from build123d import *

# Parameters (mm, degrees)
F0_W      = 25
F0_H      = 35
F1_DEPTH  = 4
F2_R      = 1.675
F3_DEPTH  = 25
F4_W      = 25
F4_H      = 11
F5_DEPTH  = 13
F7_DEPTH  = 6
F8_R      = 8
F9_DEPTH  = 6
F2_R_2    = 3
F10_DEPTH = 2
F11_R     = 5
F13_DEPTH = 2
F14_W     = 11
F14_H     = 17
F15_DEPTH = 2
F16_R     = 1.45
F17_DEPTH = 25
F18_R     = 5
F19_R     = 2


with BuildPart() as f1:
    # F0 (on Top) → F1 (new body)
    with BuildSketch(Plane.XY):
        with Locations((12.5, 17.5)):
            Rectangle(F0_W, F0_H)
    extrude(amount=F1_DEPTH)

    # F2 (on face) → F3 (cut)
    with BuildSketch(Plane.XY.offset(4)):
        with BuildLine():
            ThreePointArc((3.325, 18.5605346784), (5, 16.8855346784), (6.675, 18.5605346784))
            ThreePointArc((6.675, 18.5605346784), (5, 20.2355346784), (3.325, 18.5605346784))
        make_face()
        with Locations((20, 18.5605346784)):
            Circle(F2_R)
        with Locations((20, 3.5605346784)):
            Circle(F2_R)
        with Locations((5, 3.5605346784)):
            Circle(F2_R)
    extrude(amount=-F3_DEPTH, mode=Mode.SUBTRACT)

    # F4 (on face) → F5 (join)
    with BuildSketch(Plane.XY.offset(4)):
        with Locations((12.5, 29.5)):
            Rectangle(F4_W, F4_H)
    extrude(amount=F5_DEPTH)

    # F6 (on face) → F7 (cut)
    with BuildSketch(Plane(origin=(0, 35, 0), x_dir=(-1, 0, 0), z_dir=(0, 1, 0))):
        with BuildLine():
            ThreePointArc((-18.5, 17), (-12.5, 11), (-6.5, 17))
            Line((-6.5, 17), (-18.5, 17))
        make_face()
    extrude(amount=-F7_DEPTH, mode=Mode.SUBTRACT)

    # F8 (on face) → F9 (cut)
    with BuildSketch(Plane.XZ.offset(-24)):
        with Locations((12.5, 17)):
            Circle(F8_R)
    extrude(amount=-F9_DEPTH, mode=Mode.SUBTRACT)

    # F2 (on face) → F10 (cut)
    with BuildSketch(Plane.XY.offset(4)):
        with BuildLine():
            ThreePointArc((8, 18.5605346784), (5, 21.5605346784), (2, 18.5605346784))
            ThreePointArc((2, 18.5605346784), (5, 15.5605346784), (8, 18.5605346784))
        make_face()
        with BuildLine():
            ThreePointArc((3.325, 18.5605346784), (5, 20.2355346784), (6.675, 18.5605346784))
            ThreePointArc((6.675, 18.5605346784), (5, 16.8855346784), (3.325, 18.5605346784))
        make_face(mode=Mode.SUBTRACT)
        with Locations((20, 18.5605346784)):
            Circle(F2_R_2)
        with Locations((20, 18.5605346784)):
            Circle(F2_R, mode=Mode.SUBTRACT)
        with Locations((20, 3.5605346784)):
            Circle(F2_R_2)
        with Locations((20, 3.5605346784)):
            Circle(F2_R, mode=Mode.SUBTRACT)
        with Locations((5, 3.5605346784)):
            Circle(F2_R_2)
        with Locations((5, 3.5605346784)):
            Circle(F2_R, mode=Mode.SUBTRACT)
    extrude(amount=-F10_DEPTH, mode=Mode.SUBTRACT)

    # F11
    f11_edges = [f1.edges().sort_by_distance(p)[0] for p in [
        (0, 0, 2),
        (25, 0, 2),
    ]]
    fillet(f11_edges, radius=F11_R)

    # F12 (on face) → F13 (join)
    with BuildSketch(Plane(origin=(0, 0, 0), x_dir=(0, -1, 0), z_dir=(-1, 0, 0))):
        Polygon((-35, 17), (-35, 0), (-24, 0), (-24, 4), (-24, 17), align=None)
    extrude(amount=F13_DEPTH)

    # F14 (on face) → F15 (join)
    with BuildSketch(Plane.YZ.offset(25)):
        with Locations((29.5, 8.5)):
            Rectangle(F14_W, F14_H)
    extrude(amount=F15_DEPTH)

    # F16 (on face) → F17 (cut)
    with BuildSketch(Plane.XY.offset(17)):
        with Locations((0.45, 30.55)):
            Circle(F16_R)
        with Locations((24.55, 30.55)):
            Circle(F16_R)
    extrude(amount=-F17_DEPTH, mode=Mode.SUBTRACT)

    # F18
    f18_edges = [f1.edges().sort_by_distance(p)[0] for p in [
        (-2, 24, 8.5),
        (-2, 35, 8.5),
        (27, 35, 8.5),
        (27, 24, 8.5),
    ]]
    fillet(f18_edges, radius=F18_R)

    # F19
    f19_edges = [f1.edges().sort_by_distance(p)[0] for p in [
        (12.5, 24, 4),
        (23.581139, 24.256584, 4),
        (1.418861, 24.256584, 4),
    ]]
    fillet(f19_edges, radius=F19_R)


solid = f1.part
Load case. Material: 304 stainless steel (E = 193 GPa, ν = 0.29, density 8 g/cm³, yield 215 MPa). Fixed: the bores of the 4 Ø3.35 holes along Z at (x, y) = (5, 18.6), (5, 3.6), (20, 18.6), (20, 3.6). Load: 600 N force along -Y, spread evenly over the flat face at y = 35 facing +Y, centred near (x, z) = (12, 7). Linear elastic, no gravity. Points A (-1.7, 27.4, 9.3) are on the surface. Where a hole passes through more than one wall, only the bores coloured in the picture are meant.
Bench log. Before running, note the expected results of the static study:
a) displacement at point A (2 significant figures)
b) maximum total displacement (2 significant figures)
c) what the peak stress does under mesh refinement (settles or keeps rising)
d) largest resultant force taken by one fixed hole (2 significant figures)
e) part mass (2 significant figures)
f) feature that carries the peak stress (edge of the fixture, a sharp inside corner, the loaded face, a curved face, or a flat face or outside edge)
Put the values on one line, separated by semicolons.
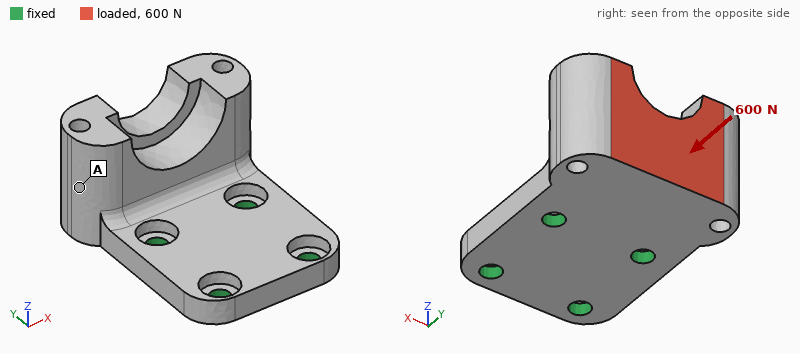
13 µm; 27 µm; keeps rising; 220 N; 48 g; edge of the fixture
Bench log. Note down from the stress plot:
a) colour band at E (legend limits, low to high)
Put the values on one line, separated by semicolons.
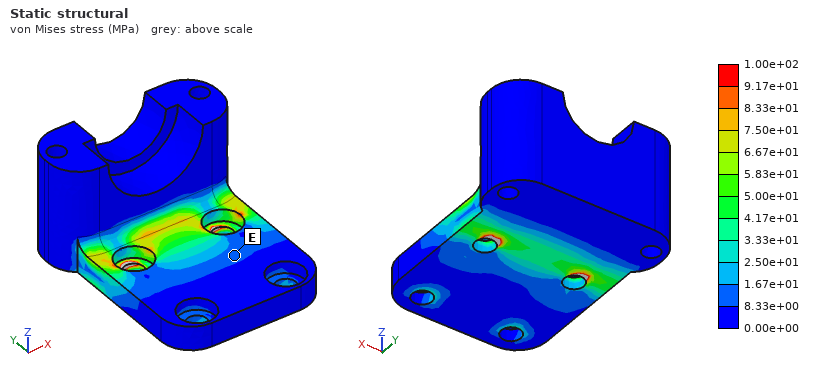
8.33e+00 to 1.67e+01 MPa
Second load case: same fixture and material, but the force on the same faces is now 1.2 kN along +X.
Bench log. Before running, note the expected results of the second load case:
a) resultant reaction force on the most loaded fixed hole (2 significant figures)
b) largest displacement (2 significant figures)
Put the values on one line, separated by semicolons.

1.3 kN; 8.9 µm
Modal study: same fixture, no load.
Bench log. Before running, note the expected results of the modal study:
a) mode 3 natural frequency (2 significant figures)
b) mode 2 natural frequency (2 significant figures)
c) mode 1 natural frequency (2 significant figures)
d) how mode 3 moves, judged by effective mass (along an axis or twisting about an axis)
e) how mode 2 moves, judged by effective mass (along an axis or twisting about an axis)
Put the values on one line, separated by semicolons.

16 kHz; 10 kHz; 3900 Hz; along X; along X
